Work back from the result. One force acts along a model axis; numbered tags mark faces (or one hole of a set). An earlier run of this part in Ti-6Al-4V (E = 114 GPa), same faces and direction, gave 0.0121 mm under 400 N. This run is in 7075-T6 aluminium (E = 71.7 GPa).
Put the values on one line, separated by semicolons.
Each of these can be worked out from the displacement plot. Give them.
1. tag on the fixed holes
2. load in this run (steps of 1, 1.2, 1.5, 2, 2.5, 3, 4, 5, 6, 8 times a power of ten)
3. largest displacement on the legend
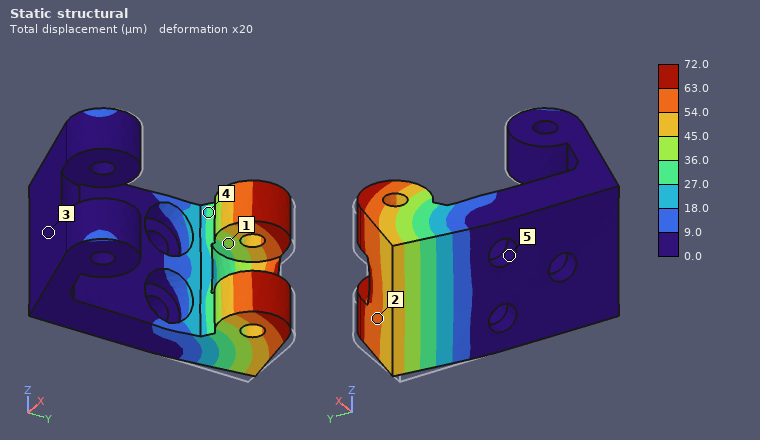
5; 1.5 kN; 72.0 µm
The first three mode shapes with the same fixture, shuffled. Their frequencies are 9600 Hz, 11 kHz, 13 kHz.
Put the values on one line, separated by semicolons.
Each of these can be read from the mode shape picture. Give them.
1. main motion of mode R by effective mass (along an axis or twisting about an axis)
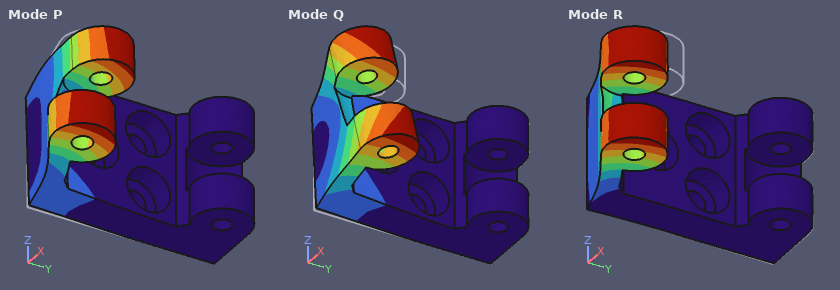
along Y
